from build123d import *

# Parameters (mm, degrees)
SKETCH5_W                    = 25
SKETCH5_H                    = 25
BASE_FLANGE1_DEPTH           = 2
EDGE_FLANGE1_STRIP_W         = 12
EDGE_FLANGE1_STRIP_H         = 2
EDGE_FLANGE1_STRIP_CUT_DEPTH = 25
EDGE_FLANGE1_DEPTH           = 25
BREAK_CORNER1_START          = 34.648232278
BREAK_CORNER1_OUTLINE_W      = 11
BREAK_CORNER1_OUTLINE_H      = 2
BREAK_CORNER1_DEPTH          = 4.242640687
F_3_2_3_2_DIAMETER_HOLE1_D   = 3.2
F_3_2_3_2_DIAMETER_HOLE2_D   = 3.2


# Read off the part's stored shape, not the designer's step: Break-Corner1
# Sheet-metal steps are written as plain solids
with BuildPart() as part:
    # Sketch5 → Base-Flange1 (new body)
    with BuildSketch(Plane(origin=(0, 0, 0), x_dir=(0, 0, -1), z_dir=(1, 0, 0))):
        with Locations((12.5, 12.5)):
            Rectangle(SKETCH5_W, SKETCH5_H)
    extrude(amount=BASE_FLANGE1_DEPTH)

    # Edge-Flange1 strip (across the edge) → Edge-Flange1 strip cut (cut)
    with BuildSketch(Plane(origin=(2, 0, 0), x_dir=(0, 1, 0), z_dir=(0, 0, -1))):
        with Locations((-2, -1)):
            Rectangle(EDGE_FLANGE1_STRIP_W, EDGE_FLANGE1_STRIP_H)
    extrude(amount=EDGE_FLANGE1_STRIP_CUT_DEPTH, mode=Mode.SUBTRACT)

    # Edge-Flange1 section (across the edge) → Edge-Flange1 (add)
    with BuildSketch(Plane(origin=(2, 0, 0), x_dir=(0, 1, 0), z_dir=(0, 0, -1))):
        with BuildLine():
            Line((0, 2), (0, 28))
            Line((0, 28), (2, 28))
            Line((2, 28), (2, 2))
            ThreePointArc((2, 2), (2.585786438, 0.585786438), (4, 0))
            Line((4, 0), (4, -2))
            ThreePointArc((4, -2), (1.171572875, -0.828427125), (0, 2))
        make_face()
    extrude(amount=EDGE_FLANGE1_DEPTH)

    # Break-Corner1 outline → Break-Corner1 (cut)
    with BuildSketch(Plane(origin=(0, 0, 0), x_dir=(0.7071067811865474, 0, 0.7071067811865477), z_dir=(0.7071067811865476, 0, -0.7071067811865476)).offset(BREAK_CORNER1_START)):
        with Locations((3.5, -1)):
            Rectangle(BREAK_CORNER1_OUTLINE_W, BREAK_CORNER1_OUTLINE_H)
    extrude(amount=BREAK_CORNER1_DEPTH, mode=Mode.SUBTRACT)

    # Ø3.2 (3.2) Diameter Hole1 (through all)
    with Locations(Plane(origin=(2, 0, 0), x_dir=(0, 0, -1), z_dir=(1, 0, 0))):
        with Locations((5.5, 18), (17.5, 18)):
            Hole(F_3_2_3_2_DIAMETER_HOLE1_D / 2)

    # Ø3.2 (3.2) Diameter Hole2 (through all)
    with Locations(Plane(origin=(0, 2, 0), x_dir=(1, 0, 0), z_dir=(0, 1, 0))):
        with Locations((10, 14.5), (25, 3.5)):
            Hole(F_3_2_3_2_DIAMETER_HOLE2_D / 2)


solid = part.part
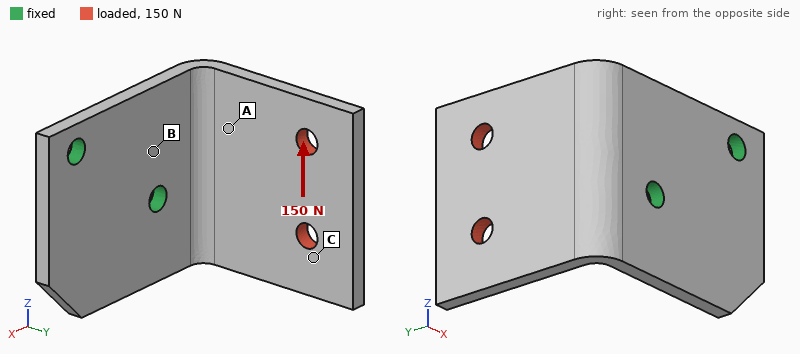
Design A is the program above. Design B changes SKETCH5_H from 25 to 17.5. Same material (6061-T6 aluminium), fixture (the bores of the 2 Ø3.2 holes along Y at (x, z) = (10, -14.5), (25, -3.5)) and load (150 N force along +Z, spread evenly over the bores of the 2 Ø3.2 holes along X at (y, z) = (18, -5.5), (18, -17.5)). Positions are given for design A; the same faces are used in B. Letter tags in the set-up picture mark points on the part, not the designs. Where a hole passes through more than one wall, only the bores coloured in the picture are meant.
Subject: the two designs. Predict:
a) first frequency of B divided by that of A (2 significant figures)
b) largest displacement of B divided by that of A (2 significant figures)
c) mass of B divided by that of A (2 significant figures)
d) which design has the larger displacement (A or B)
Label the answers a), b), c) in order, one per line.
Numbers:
a) 1.3
b) 0.89
c) 0.92
d) A
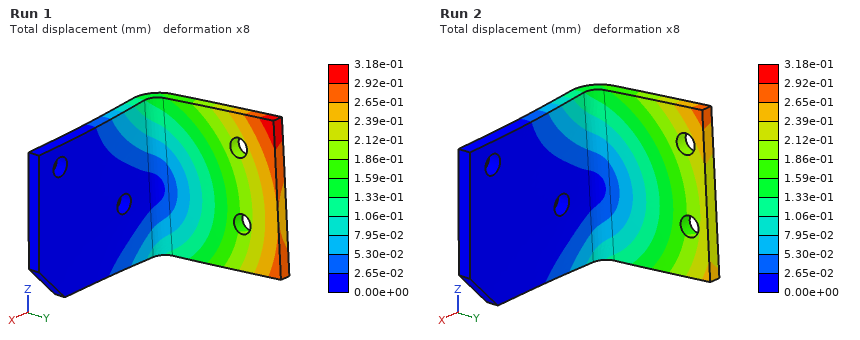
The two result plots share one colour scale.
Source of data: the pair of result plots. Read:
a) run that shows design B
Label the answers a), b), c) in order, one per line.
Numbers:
a) Run 2
